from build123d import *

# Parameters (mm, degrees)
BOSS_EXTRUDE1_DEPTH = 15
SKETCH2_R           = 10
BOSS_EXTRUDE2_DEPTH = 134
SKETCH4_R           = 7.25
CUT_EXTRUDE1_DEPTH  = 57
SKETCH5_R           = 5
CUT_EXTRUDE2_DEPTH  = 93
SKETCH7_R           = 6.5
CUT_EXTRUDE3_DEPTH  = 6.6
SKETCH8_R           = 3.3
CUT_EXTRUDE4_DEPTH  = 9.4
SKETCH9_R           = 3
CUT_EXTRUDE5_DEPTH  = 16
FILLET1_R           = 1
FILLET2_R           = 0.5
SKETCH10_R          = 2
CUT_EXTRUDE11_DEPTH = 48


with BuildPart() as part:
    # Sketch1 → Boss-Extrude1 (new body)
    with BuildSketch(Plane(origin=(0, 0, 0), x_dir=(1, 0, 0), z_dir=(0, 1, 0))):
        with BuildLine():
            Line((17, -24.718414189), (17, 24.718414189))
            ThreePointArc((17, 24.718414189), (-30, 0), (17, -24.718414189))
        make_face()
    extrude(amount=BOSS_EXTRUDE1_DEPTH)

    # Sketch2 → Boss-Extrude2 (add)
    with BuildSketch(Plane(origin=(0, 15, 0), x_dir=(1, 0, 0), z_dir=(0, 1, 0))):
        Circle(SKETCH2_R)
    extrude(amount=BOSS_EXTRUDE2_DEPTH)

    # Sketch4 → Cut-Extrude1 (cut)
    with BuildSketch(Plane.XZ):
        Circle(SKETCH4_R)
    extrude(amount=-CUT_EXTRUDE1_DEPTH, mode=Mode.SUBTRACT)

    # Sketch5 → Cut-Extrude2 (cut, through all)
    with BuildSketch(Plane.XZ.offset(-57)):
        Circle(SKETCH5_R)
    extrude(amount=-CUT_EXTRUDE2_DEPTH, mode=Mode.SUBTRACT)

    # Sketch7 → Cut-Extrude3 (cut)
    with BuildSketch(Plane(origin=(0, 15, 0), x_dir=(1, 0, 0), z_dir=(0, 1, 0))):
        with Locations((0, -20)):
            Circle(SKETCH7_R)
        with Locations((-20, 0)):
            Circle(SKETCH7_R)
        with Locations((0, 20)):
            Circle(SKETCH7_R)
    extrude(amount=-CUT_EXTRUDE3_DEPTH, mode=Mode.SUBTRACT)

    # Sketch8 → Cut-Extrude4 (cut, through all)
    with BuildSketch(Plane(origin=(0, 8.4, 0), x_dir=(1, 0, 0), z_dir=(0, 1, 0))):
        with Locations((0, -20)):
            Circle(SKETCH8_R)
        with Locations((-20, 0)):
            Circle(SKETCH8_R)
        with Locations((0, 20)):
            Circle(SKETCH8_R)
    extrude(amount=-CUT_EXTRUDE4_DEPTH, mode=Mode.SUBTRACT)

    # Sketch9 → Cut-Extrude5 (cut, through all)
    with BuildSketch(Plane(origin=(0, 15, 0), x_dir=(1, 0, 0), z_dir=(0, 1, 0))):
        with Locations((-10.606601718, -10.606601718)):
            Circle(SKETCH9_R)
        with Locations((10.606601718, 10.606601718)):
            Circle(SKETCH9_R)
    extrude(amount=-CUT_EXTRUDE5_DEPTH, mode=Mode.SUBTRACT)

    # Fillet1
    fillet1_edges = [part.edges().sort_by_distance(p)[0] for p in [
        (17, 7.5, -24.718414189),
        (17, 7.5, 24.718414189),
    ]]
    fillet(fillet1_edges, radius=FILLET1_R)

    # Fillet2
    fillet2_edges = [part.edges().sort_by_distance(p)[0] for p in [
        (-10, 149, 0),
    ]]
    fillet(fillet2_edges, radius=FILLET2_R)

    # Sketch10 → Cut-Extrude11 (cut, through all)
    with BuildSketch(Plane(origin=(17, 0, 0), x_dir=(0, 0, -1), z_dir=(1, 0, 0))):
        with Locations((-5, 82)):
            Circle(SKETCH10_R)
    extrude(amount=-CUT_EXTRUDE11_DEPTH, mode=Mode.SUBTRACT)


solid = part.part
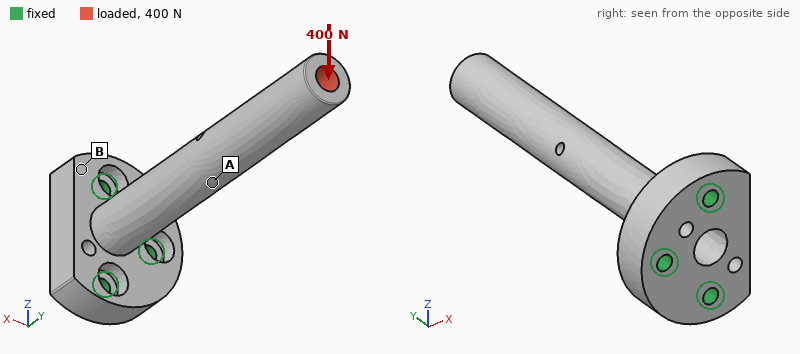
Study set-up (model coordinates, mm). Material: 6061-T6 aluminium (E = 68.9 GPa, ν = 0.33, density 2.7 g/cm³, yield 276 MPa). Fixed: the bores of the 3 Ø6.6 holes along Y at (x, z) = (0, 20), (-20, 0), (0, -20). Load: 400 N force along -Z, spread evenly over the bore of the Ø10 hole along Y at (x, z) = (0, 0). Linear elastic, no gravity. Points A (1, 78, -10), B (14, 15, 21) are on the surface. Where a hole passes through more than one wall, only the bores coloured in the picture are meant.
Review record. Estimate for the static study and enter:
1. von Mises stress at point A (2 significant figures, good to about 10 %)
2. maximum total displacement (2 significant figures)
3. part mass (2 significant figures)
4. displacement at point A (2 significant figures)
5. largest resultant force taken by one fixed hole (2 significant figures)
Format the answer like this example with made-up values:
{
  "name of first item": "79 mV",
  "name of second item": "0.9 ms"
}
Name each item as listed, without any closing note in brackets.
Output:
{
  "von Mises stress at point A": "16 MPa",
  "maximum total displacement": "0.50 mm",
  "part mass": "150 g",
  "displacement at point A": "0.18 mm",
  "largest resultant force taken by one fixed hole": "1.1 kN"
}
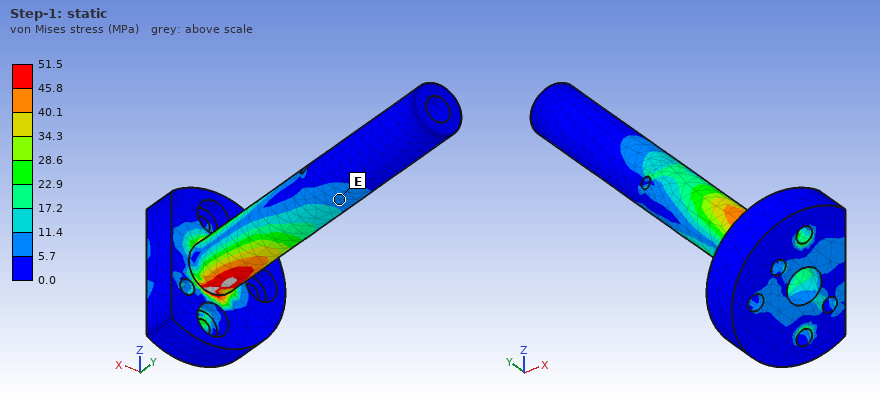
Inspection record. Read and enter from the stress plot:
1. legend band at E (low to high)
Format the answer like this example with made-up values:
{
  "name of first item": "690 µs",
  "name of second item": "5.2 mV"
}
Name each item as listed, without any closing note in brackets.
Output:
{
  "legend band at E": "5.7 to 11.4 MPa"
}
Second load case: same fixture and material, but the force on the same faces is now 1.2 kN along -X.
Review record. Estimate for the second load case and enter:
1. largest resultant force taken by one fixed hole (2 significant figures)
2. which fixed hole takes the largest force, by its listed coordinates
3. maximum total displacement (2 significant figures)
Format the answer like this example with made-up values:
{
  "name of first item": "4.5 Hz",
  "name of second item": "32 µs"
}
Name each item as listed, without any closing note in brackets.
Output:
{
  "largest resultant force taken by one fixed hole": "4.3 kN",
  "which fixed hole takes the largest force, by its listed coordinates": "(-20, 0)",
  "maximum total displacement": "1.6 mm"
}
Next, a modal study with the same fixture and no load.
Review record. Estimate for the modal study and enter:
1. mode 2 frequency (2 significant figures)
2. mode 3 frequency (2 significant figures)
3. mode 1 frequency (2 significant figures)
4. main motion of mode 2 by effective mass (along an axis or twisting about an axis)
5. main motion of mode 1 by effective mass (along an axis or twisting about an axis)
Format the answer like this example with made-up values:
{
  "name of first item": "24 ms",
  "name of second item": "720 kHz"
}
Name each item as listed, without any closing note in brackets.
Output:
{
  "mode 2 frequency": "710 Hz",
  "mode 3 frequency": "4200 Hz",
  "mode 1 frequency": "680 Hz",
  "main motion of mode 2 by effective mass": "along Z",
  "main motion of mode 1 by effective mass": "along X"
}
